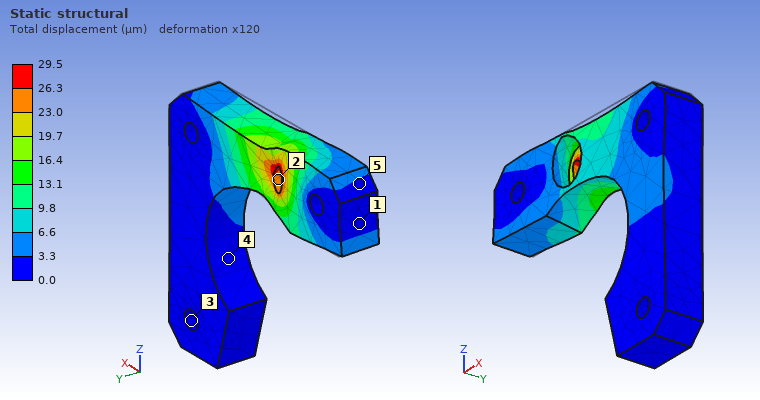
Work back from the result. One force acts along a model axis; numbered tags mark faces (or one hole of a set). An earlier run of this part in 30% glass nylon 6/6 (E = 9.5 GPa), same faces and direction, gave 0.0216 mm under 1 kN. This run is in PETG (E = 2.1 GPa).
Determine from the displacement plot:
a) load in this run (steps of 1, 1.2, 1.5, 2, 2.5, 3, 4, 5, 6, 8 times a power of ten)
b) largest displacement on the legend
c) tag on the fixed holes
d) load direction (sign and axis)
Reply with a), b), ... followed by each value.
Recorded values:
a) 300 N
b) 29.5 µm
c) 3
d) -X
